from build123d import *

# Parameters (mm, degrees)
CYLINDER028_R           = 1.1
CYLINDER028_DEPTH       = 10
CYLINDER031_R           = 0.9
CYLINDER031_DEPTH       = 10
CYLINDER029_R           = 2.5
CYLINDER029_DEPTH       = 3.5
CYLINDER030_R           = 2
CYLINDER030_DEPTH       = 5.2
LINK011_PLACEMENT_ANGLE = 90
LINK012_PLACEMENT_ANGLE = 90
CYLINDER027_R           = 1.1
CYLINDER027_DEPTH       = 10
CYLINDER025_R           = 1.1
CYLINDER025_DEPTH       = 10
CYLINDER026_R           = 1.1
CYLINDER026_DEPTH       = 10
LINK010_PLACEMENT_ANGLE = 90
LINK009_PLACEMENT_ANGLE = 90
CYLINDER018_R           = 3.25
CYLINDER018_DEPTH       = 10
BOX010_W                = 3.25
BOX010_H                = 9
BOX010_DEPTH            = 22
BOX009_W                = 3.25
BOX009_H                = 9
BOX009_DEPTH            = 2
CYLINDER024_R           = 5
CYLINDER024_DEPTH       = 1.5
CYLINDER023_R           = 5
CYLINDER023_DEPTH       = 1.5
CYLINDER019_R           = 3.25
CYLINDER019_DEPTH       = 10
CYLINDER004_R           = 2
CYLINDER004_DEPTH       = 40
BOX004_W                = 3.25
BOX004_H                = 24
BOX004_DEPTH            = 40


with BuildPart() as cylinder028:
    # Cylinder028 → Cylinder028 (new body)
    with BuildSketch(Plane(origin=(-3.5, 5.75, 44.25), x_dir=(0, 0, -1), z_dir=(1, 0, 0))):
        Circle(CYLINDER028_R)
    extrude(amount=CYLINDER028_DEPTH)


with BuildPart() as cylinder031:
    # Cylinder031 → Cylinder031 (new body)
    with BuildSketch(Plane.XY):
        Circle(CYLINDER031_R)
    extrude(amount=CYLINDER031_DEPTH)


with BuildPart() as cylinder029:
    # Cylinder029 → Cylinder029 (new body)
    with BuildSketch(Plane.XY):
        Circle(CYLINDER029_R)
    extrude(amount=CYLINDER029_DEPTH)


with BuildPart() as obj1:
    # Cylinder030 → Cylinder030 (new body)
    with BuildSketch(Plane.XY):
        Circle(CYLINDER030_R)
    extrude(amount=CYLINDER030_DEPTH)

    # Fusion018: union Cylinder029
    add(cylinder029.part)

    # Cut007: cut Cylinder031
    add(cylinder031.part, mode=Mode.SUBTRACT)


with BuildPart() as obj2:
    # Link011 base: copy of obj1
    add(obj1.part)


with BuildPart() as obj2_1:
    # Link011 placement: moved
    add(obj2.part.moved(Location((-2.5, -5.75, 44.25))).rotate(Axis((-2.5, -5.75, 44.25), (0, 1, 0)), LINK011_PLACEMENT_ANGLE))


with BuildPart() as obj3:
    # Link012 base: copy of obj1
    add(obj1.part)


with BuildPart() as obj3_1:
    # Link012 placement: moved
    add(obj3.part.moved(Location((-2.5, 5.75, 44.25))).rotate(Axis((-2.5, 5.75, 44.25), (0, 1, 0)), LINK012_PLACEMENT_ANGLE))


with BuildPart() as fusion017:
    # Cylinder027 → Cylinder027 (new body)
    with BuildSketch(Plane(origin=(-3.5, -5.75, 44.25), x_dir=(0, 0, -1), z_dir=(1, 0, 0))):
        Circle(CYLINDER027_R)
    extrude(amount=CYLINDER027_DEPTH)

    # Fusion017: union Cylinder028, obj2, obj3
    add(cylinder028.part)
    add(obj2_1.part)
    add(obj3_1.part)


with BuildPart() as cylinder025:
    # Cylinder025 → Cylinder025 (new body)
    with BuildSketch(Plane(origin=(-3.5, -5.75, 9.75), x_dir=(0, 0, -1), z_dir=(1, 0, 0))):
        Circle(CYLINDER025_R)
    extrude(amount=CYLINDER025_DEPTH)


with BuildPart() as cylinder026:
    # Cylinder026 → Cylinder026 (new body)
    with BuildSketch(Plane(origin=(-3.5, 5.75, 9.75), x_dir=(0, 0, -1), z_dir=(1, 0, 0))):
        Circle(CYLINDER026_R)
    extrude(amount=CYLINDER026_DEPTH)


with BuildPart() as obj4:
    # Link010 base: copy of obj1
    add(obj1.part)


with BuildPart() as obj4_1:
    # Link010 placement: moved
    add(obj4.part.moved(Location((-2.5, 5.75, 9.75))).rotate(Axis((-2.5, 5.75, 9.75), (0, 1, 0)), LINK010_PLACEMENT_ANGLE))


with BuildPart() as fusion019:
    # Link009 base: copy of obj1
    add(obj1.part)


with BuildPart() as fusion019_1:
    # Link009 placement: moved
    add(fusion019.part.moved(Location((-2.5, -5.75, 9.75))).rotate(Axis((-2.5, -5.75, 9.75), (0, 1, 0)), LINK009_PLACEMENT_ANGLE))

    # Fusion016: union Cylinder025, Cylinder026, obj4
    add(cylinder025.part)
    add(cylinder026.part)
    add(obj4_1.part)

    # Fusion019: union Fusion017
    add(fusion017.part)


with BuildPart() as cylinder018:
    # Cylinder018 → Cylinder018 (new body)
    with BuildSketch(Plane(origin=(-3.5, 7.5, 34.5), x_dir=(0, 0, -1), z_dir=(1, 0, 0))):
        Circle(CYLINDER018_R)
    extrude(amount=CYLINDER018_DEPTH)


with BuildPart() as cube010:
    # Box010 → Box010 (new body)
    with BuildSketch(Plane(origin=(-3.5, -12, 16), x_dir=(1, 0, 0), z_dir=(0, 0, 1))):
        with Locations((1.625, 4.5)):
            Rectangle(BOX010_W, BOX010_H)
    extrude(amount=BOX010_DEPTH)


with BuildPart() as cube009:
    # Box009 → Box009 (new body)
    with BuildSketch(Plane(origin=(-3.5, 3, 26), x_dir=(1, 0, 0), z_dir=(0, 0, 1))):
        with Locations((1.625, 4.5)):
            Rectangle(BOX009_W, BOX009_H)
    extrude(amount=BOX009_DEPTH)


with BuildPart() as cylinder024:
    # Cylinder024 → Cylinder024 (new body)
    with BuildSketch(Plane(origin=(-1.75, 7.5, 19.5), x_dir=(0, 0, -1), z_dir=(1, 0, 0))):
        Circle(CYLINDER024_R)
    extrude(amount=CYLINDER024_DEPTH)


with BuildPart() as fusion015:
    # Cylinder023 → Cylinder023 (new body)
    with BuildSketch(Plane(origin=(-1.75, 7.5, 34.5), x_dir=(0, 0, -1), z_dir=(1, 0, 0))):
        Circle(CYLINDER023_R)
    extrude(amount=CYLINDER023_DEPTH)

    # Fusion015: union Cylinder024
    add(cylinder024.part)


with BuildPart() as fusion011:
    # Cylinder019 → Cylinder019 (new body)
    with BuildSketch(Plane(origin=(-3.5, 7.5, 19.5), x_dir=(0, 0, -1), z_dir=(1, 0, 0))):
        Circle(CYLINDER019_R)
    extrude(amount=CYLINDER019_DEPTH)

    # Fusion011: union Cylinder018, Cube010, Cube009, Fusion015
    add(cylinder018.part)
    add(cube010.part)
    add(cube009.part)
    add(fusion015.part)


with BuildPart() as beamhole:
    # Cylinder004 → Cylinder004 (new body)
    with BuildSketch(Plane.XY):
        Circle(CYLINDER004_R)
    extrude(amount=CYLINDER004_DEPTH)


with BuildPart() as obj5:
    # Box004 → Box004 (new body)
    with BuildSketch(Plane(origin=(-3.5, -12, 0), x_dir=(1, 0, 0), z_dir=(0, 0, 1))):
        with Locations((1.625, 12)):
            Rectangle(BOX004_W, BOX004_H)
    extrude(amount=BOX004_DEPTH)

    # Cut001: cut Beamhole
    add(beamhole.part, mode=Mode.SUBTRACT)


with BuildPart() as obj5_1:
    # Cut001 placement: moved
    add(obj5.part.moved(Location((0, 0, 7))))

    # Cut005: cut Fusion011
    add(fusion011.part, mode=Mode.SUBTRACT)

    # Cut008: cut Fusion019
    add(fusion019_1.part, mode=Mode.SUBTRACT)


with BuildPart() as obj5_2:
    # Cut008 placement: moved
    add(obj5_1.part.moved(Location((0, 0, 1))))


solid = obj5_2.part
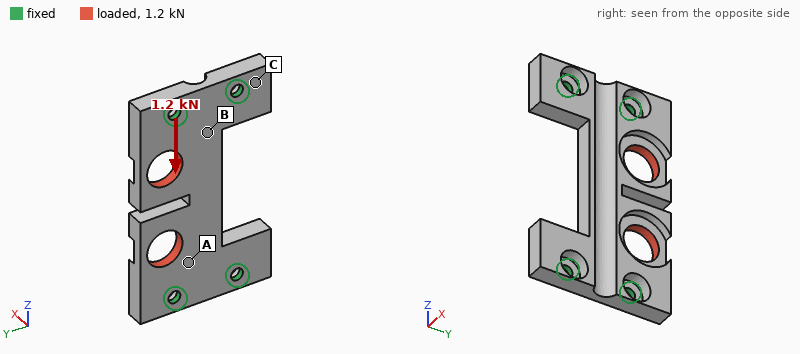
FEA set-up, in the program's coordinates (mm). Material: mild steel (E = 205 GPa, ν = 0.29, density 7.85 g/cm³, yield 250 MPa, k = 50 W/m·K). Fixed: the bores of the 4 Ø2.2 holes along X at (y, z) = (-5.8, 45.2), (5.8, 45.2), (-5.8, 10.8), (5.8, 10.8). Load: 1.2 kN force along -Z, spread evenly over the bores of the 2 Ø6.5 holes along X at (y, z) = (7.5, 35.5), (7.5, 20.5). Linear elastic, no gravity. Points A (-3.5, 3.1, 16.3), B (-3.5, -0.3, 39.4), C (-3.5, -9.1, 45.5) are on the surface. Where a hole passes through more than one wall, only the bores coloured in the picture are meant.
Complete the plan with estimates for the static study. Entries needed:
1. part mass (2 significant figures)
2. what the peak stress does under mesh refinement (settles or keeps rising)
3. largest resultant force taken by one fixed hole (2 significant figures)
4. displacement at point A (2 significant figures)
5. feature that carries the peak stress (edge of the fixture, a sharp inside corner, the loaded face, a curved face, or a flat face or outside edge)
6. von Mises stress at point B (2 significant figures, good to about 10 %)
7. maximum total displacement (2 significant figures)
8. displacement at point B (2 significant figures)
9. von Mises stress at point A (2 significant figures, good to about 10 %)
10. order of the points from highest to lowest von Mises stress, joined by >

13 g
keeps rising
490 N
1.6 µm
edge of the fixture
23 MPa
4.9 µm
1.4 µm
35 MPa
A > B > C
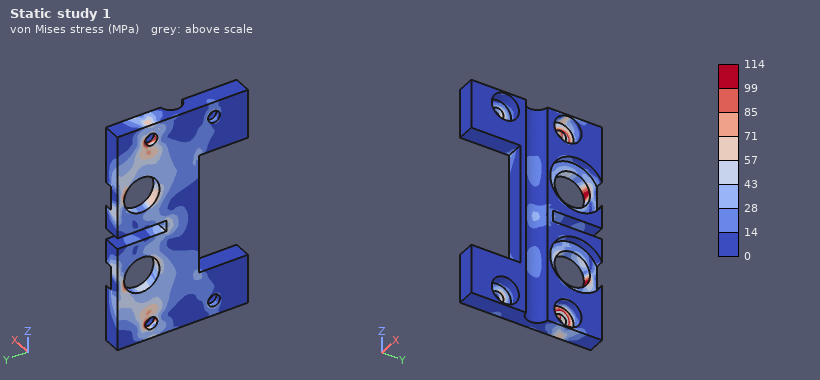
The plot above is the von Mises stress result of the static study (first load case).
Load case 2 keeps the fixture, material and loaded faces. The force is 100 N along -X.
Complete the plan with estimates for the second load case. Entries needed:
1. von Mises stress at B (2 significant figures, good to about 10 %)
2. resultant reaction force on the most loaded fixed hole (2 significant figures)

14 MPa
66 N
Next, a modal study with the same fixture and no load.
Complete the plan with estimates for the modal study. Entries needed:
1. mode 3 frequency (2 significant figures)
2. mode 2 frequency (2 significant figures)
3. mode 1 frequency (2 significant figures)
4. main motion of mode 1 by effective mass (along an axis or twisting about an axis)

15 kHz
14 kHz
7900 Hz
along X
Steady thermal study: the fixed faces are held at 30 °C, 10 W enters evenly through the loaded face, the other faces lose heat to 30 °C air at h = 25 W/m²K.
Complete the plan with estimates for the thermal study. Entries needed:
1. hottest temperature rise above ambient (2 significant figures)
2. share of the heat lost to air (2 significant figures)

52 K
9.7 %
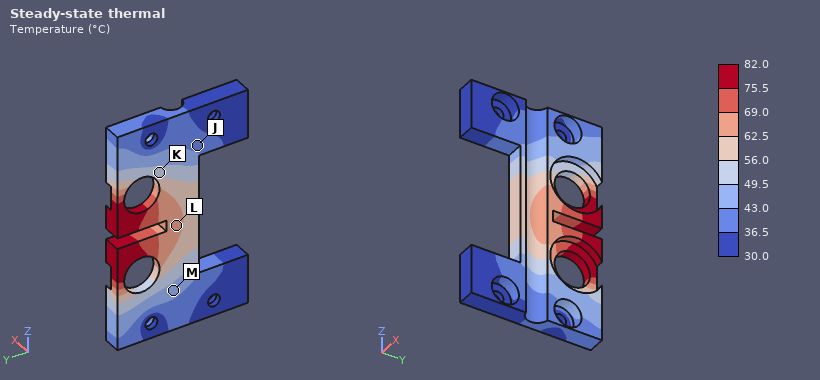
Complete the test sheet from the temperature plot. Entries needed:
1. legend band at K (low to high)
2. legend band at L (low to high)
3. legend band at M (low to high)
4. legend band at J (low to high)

49.5 to 56.0 °C
62.5 to 69.0 °C
43.0 to 49.5 °C
36.5 to 43.0 °C
